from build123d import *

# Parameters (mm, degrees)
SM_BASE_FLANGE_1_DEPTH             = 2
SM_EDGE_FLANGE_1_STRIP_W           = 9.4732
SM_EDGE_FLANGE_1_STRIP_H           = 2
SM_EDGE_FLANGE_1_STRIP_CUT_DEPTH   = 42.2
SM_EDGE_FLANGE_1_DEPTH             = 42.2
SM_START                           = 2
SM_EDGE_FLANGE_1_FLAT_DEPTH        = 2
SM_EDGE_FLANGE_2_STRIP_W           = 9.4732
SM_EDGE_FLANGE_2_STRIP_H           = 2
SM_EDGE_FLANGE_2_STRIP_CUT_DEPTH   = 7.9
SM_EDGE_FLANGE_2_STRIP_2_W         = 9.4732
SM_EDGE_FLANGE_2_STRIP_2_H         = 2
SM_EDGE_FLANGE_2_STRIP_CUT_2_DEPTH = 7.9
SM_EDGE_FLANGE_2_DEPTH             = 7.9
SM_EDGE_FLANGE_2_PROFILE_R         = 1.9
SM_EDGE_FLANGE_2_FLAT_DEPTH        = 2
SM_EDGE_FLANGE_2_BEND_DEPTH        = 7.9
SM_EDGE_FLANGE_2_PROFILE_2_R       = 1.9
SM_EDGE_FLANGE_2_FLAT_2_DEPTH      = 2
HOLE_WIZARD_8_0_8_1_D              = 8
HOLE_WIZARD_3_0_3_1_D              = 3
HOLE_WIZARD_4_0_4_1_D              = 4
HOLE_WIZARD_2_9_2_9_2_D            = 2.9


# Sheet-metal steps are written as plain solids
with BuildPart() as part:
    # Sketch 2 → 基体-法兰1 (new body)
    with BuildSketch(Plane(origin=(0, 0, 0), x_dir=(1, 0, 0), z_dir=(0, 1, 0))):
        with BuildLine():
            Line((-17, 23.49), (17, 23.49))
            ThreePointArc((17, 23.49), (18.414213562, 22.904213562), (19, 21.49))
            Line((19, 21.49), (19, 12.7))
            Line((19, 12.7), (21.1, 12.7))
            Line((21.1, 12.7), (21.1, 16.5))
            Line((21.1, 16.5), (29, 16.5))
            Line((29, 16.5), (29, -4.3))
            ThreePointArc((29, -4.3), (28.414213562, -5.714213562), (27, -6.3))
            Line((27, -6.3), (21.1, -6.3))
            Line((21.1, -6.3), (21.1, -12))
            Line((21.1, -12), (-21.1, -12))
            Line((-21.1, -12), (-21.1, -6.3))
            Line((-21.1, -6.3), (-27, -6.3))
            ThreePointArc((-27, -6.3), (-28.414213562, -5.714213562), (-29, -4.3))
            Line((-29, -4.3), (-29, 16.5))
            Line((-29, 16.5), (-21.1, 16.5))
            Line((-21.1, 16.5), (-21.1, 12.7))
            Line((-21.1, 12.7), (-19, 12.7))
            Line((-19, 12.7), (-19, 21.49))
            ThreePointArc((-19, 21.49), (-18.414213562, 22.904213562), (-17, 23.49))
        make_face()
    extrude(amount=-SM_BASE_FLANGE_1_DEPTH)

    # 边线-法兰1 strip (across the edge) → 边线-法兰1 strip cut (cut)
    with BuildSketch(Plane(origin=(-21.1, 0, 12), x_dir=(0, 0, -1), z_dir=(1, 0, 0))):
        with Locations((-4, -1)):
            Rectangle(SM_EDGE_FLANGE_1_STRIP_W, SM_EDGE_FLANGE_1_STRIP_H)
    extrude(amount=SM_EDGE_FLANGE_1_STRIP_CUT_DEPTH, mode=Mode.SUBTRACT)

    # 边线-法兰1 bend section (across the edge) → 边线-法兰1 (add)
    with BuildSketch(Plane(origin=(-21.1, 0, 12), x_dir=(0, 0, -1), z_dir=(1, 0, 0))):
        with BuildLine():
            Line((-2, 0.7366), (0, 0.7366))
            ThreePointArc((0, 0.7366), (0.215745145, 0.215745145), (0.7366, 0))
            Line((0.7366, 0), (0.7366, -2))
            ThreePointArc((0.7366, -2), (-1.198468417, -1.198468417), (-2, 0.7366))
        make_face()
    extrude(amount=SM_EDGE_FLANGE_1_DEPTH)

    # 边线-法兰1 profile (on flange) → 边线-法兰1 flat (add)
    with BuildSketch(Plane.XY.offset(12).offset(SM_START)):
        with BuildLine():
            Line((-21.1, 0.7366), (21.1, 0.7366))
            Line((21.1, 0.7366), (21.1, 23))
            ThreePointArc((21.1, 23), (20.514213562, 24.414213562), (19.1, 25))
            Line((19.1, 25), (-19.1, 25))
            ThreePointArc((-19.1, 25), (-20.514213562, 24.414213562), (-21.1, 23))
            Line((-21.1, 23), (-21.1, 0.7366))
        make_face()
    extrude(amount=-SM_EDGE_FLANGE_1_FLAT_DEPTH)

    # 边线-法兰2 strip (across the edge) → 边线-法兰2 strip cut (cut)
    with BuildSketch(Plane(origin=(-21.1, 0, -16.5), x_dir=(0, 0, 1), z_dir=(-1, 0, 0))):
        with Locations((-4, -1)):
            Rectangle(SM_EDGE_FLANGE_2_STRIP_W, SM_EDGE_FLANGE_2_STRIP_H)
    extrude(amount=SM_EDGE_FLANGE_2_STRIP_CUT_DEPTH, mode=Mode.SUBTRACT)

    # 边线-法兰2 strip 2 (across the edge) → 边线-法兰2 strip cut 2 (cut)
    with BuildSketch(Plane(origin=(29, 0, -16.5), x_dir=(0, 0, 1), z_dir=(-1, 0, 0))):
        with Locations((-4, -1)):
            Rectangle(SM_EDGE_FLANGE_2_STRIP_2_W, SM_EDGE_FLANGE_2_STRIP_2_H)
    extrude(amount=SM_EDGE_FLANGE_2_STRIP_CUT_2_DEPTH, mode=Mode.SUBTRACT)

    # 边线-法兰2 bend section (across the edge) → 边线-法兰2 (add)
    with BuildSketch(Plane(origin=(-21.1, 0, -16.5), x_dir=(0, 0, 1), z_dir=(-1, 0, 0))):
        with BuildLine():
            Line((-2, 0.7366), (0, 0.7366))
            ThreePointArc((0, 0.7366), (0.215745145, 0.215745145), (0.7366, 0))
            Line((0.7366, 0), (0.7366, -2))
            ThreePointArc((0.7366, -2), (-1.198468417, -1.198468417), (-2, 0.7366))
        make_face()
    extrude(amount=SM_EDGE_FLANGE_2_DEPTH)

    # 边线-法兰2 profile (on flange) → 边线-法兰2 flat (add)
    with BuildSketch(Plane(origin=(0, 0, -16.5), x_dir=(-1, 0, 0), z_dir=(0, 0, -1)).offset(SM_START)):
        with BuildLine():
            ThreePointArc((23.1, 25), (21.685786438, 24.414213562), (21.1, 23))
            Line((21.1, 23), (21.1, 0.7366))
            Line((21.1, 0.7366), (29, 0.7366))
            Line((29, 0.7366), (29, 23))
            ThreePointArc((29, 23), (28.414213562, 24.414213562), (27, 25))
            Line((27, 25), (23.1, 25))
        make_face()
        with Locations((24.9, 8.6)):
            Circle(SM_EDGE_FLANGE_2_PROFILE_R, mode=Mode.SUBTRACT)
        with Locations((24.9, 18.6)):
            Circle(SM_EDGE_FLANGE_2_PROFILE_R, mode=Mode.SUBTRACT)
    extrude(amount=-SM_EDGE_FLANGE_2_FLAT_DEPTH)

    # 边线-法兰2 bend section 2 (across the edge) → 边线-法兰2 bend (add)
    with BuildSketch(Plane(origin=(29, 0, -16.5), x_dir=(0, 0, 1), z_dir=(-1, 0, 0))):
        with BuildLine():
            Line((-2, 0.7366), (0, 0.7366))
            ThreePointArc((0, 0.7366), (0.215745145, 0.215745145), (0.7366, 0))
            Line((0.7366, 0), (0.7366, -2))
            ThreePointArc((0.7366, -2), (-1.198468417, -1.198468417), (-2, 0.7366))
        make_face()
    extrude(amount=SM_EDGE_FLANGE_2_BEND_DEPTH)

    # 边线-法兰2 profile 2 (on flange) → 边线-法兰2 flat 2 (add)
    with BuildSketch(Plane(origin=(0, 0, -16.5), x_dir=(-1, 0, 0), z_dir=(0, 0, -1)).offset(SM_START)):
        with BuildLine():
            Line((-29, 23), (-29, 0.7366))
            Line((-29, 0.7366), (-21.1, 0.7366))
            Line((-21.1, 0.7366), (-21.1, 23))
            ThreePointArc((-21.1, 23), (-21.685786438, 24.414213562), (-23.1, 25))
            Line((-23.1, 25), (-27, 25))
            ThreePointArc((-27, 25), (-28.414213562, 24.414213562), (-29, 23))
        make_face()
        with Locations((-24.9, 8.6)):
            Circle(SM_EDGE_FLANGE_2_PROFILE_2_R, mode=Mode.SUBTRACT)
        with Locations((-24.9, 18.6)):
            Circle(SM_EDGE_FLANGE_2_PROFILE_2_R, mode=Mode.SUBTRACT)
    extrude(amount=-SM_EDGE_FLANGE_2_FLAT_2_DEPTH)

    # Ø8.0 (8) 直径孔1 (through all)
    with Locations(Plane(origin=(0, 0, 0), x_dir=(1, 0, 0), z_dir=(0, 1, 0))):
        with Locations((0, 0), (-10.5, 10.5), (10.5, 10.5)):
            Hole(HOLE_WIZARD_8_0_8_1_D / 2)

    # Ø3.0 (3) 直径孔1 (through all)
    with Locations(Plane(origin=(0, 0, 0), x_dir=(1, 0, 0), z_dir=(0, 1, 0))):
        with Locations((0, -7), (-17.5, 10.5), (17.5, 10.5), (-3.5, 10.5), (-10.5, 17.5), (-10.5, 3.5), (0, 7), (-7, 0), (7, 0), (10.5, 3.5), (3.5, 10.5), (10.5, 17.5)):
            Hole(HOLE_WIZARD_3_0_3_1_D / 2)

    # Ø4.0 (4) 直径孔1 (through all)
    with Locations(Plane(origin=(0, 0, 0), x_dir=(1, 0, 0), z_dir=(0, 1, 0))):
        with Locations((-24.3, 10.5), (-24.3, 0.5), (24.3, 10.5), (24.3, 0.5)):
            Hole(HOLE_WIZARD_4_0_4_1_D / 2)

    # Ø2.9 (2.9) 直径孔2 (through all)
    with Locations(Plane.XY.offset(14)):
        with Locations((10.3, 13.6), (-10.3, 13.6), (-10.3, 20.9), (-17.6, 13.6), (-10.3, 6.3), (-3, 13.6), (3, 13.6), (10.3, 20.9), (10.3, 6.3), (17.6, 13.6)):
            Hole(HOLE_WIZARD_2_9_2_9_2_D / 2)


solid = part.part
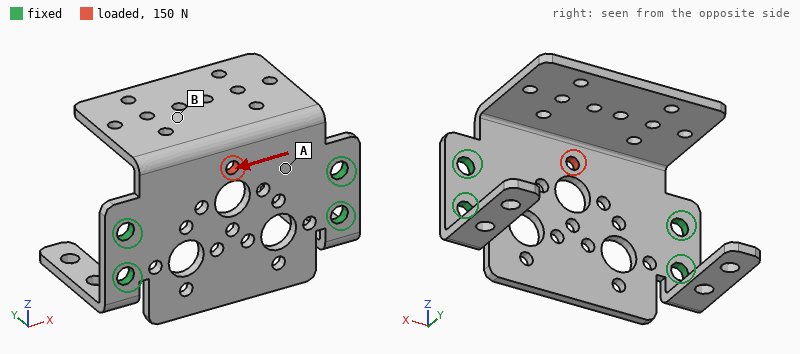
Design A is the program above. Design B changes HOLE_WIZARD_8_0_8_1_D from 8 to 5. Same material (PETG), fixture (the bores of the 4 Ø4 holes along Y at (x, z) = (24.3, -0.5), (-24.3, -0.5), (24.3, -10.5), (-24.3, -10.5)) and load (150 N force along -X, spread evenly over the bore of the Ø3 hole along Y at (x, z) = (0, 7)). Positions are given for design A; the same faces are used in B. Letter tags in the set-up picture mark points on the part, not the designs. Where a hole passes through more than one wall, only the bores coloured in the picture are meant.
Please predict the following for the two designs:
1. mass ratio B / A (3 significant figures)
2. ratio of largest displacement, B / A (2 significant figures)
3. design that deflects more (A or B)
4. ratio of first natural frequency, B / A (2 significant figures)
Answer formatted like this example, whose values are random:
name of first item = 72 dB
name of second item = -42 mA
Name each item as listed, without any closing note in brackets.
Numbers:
mass ratio B / A = 1.03
ratio of largest displacement, B / A = 0.91
design that deflects more = A
ratio of first natural frequency, B / A = 1.0
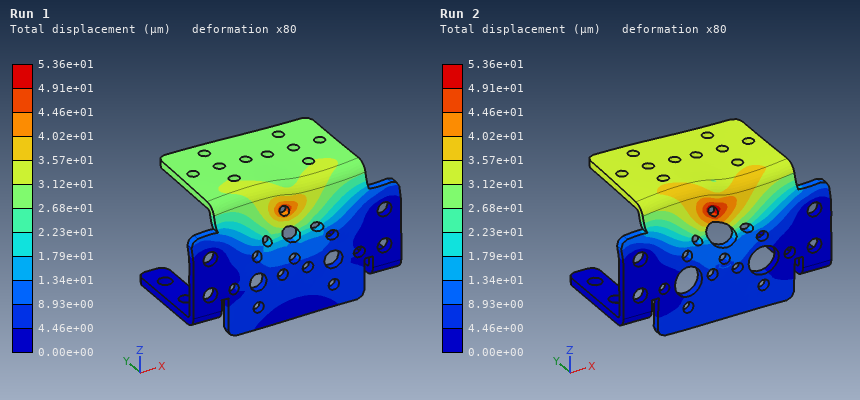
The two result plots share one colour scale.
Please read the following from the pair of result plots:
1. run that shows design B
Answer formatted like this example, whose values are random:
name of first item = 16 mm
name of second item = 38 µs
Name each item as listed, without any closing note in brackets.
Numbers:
run that shows design B = Run 1
